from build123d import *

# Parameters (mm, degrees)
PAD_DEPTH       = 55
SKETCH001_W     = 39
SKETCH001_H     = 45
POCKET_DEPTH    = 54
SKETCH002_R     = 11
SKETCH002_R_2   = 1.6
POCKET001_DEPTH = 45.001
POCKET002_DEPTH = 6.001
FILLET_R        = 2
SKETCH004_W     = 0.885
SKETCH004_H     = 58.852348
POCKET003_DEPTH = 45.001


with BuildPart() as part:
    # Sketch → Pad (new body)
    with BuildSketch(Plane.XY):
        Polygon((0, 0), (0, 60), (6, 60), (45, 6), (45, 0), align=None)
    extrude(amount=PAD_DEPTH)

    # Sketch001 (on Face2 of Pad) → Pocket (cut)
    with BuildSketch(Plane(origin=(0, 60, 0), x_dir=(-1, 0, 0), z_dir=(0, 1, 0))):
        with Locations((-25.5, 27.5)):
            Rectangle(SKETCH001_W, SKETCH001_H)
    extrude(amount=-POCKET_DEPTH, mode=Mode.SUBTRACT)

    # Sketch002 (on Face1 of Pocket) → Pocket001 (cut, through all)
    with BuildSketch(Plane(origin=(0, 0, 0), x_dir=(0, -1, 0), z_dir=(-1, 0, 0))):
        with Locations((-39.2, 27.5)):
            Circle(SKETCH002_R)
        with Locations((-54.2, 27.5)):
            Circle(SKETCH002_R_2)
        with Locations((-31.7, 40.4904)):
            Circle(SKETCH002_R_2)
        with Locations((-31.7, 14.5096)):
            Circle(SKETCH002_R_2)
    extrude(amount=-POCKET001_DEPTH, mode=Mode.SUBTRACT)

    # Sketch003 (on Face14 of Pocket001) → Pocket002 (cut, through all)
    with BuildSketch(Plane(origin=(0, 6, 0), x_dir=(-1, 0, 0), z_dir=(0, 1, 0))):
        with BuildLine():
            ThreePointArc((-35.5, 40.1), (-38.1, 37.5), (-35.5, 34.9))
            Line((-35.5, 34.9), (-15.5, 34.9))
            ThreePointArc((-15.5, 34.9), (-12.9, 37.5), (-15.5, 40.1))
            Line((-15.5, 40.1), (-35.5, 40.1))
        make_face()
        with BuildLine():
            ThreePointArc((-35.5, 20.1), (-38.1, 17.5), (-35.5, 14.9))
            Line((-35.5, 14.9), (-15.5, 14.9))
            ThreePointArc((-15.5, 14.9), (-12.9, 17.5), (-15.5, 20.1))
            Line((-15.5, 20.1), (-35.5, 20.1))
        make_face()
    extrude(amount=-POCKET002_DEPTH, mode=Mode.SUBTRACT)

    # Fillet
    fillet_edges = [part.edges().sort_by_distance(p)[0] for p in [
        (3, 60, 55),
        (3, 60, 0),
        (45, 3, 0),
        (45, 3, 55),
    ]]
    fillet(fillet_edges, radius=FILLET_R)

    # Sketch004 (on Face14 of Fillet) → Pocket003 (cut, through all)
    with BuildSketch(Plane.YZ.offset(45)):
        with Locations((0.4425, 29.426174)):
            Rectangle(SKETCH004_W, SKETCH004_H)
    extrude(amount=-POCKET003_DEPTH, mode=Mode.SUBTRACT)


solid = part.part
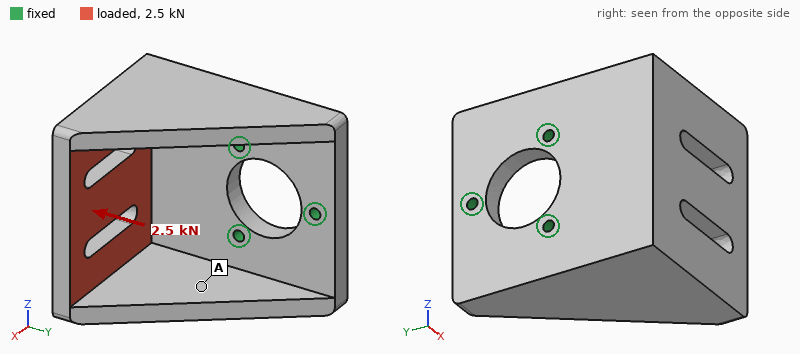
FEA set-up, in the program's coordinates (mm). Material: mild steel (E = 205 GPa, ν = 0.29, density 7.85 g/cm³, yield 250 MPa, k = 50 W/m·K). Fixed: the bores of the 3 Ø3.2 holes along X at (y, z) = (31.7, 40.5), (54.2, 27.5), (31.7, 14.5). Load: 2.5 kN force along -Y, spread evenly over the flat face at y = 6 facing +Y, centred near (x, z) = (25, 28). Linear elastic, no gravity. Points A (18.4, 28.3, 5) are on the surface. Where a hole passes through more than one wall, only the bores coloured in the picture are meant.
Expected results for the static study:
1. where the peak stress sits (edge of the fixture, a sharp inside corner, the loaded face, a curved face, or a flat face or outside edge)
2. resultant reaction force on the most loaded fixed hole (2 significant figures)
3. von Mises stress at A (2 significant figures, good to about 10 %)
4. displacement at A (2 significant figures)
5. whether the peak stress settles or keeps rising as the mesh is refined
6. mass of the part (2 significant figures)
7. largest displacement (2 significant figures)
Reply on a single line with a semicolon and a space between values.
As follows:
edge of the fixture; 1.4 kN; 21 MPa; 0.027 mm; keeps rising; 290 g; 0.11 mm
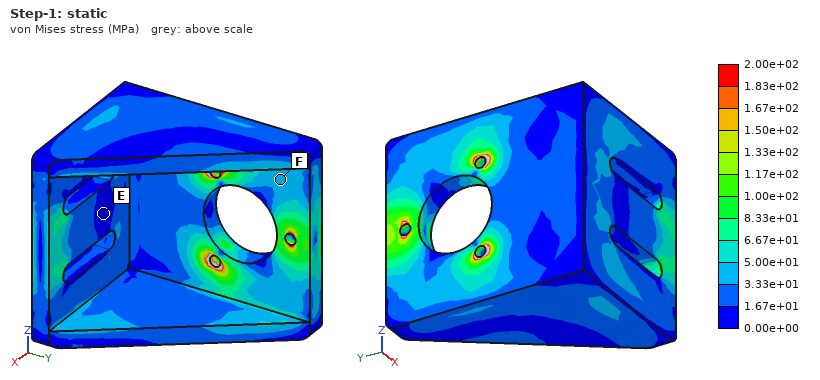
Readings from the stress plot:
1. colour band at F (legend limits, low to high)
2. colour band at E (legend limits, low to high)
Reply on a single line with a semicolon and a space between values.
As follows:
3.33e+01 to 5.00e+01 MPa; 0.00e+00 to 1.67e+01 MPa
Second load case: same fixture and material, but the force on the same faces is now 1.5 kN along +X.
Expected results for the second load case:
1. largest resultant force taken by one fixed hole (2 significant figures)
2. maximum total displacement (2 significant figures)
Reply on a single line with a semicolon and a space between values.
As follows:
1.1 kN; 53 µm
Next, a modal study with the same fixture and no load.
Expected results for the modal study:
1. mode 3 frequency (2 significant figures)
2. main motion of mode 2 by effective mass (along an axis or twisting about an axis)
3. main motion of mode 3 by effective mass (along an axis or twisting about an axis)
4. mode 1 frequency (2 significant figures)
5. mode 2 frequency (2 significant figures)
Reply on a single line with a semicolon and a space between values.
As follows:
5700 Hz; along Z; along X; 2200 Hz; 2500 Hz
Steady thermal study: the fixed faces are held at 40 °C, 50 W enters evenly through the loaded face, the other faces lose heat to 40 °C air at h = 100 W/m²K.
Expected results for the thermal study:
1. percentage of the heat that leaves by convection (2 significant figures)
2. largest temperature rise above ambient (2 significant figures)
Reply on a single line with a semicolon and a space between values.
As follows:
65 %; 67 K
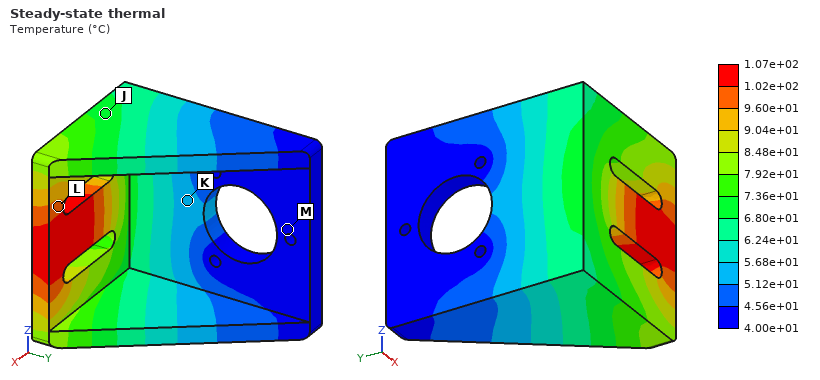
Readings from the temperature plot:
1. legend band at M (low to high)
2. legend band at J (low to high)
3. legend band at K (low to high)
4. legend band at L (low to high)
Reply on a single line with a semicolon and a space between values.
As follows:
4.00e+01 to 4.56e+01 °C; 6.80e+01 to 7.36e+01 °C; 5.12e+01 to 5.68e+01 °C; 9.60e+01 to 1.02e+02 °C
